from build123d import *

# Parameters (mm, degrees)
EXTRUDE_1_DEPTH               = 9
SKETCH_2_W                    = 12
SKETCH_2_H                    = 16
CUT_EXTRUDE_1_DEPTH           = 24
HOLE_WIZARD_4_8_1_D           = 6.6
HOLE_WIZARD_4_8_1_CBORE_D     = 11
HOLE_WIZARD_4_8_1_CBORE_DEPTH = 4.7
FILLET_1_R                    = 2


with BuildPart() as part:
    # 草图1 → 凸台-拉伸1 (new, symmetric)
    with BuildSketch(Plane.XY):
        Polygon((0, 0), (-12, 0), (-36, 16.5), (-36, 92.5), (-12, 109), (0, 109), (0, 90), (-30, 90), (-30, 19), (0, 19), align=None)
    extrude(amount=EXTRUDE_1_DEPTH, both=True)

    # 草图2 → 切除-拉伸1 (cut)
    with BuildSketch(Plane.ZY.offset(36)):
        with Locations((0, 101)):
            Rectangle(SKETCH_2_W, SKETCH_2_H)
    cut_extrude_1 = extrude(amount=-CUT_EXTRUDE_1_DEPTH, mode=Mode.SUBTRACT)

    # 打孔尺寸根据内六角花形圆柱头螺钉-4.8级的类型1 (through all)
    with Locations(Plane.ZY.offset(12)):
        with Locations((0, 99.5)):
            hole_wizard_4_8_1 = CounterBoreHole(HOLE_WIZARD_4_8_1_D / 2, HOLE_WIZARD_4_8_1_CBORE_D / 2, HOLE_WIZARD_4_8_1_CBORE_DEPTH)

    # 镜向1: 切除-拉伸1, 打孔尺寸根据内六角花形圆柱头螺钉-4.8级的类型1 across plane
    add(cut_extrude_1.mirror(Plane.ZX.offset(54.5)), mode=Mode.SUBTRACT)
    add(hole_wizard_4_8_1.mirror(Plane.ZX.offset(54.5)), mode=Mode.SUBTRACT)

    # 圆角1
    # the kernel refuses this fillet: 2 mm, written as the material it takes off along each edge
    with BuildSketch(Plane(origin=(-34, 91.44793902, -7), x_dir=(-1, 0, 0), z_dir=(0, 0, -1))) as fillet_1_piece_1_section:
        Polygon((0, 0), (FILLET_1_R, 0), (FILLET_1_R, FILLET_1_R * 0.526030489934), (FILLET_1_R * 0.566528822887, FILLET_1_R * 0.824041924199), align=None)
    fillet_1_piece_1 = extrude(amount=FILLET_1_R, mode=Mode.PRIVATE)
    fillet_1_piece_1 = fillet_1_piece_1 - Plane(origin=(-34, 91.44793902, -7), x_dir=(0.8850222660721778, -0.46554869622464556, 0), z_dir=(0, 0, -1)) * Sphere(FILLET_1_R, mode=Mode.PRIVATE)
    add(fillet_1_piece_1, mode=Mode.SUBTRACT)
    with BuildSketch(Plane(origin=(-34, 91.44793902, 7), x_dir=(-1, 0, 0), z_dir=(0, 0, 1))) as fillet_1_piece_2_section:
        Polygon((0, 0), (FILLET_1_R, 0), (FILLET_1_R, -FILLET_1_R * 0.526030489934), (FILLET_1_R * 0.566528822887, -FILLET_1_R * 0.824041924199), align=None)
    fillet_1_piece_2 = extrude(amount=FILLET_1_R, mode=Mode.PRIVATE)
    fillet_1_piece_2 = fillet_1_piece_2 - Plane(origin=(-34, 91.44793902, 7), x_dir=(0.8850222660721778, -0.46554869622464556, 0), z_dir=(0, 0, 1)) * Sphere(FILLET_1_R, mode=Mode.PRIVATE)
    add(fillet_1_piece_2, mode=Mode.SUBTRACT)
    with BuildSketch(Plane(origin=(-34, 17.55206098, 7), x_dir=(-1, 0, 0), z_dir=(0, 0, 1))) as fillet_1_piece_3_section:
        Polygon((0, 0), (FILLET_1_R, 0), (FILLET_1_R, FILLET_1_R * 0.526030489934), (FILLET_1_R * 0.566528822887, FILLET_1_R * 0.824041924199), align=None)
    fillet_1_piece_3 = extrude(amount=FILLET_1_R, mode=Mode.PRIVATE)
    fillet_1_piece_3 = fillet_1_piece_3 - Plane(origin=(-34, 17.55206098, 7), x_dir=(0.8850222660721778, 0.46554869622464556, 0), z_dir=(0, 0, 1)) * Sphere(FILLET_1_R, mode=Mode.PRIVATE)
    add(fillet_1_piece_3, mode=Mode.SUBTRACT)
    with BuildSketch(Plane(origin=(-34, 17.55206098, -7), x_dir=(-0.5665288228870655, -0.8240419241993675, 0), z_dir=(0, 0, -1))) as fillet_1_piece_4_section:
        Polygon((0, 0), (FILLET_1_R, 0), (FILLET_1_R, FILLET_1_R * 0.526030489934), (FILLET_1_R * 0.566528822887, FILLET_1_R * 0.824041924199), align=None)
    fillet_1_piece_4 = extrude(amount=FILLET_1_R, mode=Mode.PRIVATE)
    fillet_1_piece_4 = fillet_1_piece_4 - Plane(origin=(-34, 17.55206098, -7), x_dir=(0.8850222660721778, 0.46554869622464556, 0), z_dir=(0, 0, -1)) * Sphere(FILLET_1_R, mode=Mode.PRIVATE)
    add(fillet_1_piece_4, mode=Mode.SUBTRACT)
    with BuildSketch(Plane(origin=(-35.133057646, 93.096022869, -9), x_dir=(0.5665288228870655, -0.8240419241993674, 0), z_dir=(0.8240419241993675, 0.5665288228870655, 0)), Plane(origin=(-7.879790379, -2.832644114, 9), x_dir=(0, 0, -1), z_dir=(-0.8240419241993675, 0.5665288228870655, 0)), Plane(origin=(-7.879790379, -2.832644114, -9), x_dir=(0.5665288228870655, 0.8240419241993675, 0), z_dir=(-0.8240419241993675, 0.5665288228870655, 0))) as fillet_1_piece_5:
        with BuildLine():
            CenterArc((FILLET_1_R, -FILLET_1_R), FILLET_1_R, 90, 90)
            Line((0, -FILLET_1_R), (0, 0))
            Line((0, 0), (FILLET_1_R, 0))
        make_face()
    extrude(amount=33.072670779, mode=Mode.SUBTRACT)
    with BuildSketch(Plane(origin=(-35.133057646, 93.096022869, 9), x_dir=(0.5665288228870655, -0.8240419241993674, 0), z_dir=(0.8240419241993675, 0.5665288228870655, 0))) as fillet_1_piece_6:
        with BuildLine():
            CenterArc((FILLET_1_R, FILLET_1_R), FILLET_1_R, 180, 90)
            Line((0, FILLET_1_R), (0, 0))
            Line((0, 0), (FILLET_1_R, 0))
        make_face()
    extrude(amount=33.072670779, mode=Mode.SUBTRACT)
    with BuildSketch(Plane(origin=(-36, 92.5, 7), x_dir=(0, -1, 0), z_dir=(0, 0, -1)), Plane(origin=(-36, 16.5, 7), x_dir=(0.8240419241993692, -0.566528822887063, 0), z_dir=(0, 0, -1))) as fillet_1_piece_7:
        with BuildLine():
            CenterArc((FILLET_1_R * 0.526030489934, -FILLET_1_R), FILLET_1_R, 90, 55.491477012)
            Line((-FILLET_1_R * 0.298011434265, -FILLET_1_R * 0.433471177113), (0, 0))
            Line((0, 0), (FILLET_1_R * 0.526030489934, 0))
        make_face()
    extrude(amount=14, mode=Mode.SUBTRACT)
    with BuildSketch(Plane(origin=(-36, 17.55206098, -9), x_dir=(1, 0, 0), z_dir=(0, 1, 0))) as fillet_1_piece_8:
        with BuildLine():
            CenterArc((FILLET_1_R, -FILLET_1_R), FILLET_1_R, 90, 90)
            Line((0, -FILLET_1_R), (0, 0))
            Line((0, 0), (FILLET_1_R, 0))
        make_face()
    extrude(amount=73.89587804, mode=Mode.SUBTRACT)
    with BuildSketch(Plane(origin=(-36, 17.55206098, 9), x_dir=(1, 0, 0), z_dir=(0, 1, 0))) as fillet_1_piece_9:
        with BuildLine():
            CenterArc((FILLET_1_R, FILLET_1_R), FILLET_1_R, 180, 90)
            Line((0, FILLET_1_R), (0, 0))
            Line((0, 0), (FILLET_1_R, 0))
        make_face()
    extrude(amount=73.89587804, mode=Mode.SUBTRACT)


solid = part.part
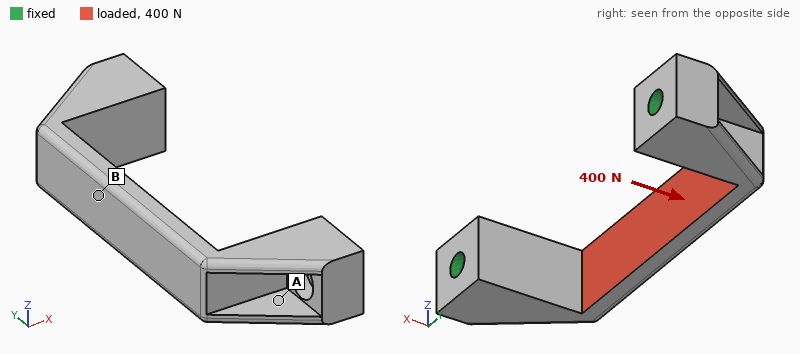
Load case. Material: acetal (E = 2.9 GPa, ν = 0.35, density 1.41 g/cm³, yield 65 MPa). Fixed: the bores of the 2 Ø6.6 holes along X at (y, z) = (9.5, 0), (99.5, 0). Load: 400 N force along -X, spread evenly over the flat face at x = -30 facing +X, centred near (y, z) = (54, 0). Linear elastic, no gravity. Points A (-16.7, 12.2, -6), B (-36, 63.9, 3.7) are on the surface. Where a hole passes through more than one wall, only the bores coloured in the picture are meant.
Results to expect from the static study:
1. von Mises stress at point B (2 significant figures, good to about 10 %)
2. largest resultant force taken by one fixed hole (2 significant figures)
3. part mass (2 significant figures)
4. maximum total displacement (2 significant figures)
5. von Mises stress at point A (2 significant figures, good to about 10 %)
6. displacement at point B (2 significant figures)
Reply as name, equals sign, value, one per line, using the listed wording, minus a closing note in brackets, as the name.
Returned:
von Mises stress at point B = 17 MPa
largest resultant force taken by one fixed hole = 250 N
part mass = 27 g
maximum total displacement = 0.98 mm
von Mises stress at point A = 4.7 MPa
displacement at point B = 0.86 mm
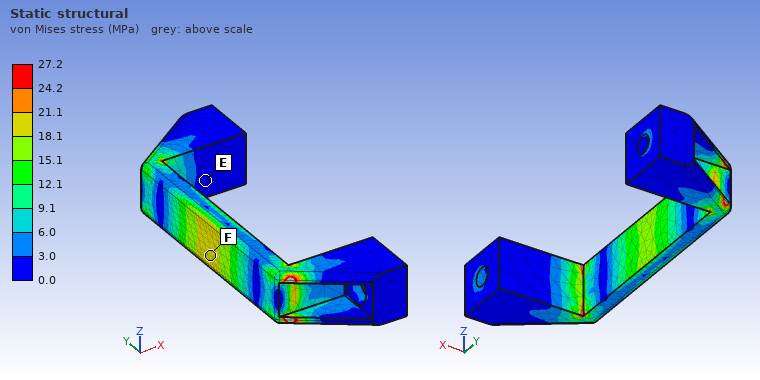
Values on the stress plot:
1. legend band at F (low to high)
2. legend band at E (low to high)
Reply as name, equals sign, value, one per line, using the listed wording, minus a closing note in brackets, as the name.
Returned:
legend band at F = 18.1 to 21.1 MPa
legend band at E = 0.0 to 3.0 MPa
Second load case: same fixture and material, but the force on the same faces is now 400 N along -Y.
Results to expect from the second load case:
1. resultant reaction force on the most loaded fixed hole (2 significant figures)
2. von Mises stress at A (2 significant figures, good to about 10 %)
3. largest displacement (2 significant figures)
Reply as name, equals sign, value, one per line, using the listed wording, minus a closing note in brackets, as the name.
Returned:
resultant reaction force on the most loaded fixed hole = 200 N
von Mises stress at A = 4.2 MPa
largest displacement = 0.35 mm
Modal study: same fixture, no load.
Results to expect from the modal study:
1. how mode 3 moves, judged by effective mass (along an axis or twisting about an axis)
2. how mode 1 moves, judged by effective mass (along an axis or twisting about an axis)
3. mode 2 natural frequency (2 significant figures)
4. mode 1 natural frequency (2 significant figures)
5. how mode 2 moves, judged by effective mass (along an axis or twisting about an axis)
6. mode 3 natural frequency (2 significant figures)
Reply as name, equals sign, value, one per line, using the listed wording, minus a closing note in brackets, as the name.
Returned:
how mode 3 moves, judged by effective mass = along Y
how mode 1 moves, judged by effective mass = along X
mode 2 natural frequency = 1300 Hz
mode 1 natural frequency = 1100 Hz
how mode 2 moves, judged by effective mass = along Z
mode 3 natural frequency = 1500 Hz
